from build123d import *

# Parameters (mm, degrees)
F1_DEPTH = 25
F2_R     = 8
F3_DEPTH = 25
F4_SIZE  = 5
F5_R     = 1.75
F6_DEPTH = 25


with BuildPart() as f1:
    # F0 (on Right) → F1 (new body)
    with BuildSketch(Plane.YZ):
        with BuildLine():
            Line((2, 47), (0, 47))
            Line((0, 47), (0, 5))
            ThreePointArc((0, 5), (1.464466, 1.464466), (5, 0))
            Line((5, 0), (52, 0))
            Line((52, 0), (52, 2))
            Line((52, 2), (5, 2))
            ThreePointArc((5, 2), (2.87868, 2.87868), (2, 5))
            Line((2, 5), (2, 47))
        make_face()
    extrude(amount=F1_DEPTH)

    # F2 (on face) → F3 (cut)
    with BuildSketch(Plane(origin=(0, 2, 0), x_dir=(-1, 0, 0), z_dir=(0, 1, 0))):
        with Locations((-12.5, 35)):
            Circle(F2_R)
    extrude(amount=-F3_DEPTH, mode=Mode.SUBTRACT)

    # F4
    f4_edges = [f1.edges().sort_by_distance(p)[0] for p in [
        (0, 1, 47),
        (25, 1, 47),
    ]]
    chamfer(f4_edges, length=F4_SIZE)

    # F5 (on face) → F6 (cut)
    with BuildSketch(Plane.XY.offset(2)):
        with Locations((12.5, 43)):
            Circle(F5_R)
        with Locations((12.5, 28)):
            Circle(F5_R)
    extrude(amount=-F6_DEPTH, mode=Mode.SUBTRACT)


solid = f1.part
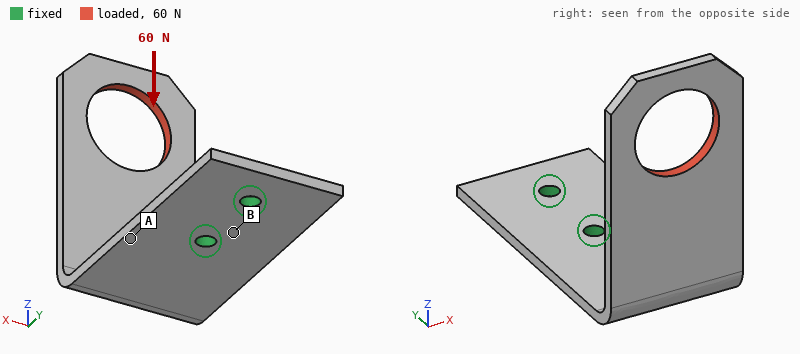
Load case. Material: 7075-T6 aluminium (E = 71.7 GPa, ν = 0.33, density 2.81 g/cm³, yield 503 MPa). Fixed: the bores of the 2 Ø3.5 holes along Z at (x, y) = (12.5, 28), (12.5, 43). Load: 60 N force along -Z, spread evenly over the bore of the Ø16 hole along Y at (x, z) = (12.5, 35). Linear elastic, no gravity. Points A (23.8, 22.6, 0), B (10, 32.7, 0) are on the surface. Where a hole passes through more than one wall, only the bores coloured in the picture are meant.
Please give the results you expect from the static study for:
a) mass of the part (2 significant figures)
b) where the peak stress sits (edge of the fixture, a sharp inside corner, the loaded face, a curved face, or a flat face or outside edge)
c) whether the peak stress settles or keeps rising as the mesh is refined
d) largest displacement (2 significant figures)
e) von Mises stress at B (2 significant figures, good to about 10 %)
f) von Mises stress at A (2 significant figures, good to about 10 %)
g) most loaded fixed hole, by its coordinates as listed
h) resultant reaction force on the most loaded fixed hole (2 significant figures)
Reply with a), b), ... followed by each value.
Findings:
a) 12 g
b) edge of the fixture
c) keeps rising
d) 0.89 mm
e) 13 MPa
f) 64 MPa
g) (12.5, 28)
h) 94 N
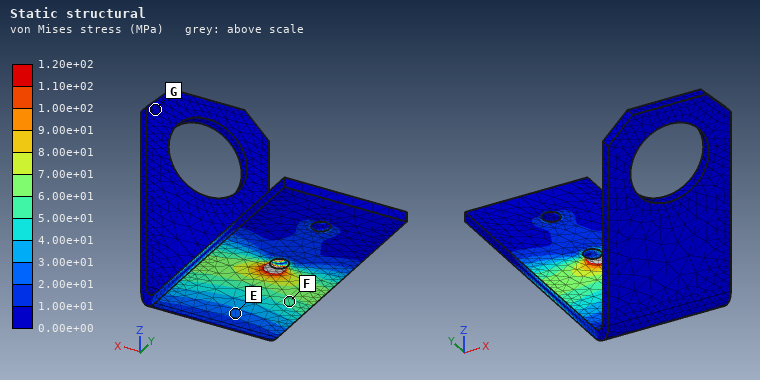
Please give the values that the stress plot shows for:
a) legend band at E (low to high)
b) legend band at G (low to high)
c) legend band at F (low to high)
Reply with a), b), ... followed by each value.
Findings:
a) 2.00e+01 to 3.00e+01 MPa
b) 0.00e+00 to 1.00e+01 MPa
c) 5.00e+01 to 6.00e+01 MPa
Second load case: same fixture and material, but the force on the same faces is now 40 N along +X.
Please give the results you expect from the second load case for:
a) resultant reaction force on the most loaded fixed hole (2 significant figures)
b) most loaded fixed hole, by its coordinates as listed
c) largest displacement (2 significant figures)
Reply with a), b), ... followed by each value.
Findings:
a) 95 N
b) (12.5, 28)
c) 0.88 mm
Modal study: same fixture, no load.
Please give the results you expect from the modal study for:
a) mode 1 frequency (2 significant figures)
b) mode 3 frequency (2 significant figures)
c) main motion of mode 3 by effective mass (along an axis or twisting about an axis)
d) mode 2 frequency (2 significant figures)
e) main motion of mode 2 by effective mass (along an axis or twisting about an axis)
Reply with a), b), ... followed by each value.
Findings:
a) 490 Hz
b) 1400 Hz
c) along Z
d) 740 Hz
e) along X
